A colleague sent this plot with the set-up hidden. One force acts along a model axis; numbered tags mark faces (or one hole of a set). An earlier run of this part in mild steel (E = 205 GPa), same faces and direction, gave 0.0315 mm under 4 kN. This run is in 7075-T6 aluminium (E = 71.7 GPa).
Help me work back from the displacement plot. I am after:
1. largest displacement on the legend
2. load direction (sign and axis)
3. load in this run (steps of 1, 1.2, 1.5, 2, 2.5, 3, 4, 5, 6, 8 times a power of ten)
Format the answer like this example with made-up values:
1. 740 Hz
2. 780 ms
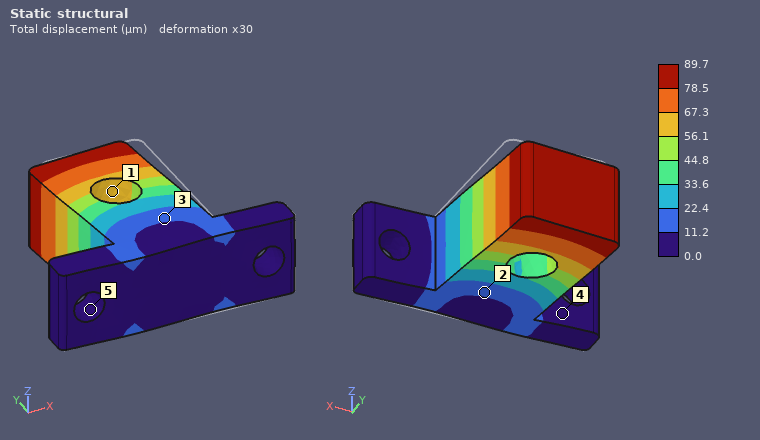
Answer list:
1. 89.7 µm
2. -X
3. 4 kN
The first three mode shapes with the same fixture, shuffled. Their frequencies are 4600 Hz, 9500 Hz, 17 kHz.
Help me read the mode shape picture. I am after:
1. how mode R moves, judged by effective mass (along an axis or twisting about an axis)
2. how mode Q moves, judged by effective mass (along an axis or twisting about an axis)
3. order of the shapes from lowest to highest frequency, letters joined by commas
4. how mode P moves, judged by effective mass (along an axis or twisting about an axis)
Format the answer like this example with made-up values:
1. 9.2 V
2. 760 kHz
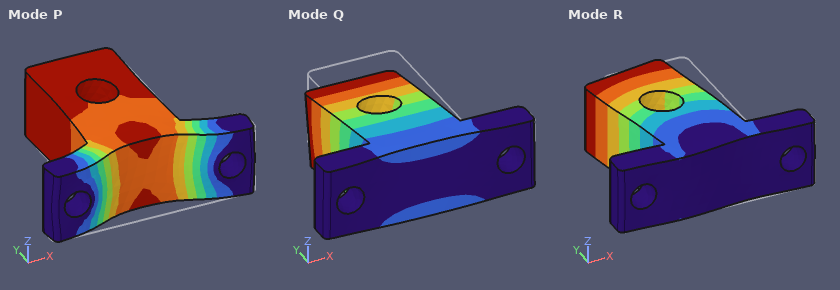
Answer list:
1. along X
2. along Z
3. Q, R, P
4. along Y
